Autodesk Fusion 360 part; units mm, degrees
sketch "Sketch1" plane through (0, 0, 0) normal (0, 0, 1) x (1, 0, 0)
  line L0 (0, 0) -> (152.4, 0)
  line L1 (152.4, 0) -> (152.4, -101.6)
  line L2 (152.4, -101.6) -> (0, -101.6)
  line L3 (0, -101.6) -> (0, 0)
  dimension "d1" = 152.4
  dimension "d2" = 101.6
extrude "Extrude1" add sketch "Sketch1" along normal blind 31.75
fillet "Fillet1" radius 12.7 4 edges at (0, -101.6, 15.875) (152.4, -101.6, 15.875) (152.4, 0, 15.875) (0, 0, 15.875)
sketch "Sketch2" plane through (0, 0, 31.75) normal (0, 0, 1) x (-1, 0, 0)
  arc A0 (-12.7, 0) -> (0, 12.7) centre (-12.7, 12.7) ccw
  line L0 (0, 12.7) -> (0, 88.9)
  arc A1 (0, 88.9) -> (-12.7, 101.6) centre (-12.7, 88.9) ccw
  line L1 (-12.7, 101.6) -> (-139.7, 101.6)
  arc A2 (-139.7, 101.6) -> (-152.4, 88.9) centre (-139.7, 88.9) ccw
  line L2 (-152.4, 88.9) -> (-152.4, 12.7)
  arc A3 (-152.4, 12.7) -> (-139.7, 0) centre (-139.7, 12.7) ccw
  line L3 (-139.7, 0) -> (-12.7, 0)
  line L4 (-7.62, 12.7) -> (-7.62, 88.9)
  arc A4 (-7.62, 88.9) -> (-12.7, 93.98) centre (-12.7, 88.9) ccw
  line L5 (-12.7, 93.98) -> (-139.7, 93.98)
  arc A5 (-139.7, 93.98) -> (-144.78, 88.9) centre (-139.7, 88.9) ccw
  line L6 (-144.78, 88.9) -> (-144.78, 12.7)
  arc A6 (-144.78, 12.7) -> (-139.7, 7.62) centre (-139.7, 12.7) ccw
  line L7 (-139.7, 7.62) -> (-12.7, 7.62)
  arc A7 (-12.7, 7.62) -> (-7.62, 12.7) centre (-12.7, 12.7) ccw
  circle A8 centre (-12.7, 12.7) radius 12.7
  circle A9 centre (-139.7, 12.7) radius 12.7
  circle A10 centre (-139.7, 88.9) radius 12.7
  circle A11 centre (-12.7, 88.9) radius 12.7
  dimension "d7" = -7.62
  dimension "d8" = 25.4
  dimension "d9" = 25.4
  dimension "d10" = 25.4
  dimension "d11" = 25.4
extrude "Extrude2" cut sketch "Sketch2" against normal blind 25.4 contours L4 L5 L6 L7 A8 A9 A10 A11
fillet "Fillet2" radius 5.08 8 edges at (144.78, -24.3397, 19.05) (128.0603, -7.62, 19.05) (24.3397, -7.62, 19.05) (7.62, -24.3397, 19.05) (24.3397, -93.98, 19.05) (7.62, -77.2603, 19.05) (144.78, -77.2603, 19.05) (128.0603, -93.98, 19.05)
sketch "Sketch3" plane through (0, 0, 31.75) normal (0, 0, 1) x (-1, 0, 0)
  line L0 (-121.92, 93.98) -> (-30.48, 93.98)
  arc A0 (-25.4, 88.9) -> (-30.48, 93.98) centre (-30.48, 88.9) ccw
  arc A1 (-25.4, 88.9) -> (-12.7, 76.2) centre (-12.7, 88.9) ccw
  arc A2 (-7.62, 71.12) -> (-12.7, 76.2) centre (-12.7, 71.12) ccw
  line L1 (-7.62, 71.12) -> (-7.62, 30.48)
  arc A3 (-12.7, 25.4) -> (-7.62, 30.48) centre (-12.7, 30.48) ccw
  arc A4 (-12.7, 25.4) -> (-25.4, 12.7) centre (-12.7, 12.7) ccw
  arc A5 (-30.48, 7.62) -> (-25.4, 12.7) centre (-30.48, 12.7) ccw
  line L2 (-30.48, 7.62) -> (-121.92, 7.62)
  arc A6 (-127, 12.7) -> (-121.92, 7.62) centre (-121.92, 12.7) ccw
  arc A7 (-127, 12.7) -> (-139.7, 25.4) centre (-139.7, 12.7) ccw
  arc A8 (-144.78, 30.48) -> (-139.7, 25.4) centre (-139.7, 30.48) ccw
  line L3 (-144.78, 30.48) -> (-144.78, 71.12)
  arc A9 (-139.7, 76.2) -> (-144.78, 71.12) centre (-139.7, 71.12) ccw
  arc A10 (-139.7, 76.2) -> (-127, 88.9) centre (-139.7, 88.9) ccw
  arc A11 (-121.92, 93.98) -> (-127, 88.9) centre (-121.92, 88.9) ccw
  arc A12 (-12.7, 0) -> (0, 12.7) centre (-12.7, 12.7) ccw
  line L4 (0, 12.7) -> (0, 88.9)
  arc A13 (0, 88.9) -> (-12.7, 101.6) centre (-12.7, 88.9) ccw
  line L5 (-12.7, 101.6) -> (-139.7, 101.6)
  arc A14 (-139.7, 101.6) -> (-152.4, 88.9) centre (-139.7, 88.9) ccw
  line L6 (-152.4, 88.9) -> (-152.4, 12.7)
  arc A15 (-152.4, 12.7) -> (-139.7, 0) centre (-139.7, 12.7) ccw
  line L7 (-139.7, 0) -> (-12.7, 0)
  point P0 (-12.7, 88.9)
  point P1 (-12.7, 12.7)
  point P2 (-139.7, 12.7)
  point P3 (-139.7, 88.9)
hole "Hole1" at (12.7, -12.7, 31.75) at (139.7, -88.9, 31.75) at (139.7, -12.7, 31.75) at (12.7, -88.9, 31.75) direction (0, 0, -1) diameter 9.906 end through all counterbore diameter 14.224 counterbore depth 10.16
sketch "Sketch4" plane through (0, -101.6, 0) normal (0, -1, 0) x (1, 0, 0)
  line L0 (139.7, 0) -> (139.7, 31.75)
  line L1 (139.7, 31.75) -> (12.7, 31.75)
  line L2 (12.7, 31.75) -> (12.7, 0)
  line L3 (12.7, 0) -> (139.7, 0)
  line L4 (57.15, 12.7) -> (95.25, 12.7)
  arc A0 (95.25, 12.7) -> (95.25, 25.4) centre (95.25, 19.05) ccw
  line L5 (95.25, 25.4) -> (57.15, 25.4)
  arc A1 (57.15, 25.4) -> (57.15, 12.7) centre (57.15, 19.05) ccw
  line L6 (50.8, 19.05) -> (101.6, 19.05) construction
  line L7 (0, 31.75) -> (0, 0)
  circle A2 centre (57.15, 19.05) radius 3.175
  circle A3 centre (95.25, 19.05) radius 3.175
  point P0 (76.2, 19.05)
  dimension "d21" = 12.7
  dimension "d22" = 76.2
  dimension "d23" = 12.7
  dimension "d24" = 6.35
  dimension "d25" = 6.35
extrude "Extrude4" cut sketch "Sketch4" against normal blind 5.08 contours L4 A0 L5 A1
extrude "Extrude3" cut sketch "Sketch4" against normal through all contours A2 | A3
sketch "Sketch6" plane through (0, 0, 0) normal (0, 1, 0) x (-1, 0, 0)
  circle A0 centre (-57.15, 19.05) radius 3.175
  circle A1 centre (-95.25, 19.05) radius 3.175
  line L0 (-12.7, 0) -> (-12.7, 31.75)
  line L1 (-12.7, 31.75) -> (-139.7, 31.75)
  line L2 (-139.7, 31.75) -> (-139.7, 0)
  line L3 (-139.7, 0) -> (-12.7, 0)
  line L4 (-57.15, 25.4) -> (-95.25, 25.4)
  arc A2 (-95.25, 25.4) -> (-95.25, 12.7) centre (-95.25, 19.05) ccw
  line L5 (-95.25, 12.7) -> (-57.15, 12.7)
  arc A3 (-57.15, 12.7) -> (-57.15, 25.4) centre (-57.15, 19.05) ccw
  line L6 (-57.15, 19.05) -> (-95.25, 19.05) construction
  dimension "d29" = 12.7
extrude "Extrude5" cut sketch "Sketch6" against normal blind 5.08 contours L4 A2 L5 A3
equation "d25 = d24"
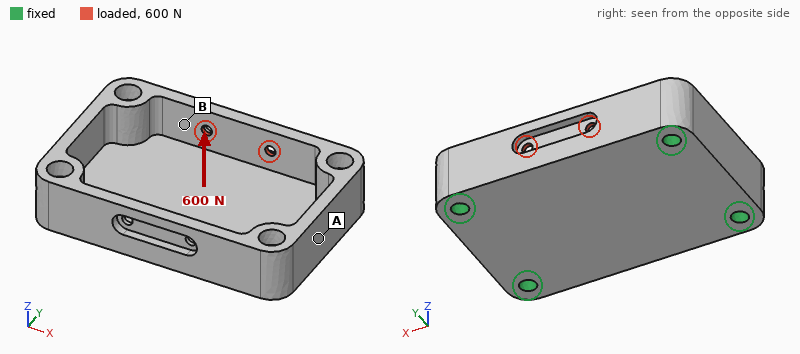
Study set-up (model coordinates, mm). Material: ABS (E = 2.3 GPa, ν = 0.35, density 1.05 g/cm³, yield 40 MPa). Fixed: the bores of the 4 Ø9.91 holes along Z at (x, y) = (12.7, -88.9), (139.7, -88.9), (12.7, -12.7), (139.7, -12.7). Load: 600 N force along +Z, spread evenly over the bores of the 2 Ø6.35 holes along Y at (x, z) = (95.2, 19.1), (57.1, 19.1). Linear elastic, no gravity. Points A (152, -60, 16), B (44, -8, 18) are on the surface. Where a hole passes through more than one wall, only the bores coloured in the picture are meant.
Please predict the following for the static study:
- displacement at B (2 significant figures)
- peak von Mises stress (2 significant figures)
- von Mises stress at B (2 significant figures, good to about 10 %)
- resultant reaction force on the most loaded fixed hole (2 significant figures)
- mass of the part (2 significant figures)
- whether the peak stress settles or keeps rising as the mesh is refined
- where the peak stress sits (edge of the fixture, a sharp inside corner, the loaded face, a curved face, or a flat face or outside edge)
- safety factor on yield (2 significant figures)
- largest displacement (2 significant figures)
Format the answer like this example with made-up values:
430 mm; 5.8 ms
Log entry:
0.096 mm; 12 MPa; 3.8 MPa; 310 N; 210 g; settles; the loaded face; 3.3; 0.18 mm
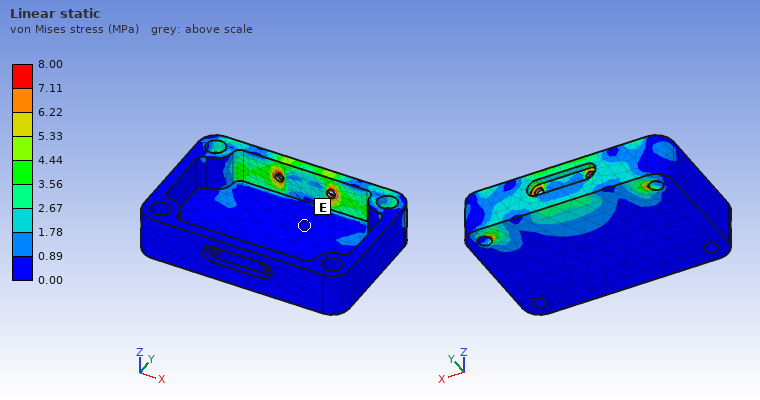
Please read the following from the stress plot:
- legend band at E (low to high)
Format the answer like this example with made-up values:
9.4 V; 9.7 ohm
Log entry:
0.00 to 0.89 MPa
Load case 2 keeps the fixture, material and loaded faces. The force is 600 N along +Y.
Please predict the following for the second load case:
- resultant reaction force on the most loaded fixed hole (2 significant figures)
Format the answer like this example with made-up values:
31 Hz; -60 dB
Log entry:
210 N
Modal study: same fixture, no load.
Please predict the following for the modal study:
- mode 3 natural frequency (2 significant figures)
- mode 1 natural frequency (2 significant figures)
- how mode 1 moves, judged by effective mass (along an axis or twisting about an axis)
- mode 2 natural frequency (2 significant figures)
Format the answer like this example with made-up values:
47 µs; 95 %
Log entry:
1900 Hz; 1000 Hz; along Z; 1800 Hz
